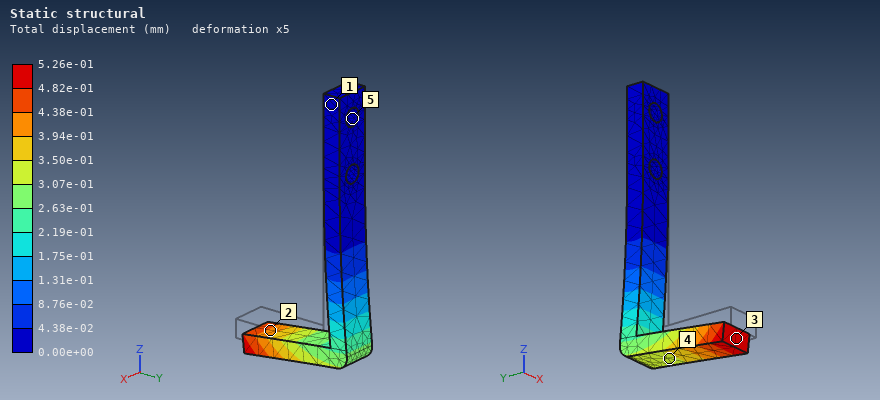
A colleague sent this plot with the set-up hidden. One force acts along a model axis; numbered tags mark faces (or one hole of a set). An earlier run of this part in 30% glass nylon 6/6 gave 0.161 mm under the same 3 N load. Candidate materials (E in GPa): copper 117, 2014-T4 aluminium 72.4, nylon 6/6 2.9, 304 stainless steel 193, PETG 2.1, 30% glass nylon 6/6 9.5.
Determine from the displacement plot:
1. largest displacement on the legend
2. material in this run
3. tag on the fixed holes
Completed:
5.26e-01 mm
nylon 6/6
5
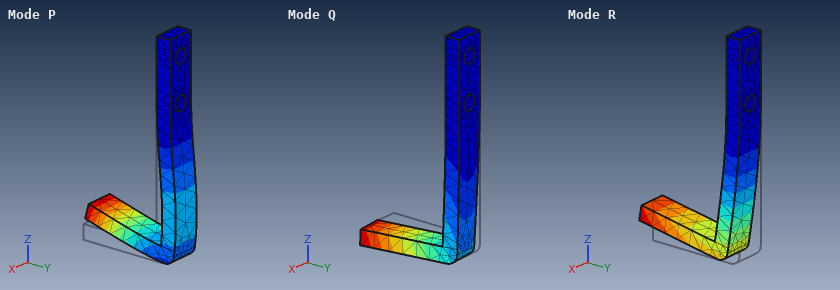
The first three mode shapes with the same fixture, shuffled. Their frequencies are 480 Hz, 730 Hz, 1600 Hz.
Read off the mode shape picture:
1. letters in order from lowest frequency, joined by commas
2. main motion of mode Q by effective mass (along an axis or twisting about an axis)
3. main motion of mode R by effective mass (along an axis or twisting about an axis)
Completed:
R, Q, P
along X
along Y
